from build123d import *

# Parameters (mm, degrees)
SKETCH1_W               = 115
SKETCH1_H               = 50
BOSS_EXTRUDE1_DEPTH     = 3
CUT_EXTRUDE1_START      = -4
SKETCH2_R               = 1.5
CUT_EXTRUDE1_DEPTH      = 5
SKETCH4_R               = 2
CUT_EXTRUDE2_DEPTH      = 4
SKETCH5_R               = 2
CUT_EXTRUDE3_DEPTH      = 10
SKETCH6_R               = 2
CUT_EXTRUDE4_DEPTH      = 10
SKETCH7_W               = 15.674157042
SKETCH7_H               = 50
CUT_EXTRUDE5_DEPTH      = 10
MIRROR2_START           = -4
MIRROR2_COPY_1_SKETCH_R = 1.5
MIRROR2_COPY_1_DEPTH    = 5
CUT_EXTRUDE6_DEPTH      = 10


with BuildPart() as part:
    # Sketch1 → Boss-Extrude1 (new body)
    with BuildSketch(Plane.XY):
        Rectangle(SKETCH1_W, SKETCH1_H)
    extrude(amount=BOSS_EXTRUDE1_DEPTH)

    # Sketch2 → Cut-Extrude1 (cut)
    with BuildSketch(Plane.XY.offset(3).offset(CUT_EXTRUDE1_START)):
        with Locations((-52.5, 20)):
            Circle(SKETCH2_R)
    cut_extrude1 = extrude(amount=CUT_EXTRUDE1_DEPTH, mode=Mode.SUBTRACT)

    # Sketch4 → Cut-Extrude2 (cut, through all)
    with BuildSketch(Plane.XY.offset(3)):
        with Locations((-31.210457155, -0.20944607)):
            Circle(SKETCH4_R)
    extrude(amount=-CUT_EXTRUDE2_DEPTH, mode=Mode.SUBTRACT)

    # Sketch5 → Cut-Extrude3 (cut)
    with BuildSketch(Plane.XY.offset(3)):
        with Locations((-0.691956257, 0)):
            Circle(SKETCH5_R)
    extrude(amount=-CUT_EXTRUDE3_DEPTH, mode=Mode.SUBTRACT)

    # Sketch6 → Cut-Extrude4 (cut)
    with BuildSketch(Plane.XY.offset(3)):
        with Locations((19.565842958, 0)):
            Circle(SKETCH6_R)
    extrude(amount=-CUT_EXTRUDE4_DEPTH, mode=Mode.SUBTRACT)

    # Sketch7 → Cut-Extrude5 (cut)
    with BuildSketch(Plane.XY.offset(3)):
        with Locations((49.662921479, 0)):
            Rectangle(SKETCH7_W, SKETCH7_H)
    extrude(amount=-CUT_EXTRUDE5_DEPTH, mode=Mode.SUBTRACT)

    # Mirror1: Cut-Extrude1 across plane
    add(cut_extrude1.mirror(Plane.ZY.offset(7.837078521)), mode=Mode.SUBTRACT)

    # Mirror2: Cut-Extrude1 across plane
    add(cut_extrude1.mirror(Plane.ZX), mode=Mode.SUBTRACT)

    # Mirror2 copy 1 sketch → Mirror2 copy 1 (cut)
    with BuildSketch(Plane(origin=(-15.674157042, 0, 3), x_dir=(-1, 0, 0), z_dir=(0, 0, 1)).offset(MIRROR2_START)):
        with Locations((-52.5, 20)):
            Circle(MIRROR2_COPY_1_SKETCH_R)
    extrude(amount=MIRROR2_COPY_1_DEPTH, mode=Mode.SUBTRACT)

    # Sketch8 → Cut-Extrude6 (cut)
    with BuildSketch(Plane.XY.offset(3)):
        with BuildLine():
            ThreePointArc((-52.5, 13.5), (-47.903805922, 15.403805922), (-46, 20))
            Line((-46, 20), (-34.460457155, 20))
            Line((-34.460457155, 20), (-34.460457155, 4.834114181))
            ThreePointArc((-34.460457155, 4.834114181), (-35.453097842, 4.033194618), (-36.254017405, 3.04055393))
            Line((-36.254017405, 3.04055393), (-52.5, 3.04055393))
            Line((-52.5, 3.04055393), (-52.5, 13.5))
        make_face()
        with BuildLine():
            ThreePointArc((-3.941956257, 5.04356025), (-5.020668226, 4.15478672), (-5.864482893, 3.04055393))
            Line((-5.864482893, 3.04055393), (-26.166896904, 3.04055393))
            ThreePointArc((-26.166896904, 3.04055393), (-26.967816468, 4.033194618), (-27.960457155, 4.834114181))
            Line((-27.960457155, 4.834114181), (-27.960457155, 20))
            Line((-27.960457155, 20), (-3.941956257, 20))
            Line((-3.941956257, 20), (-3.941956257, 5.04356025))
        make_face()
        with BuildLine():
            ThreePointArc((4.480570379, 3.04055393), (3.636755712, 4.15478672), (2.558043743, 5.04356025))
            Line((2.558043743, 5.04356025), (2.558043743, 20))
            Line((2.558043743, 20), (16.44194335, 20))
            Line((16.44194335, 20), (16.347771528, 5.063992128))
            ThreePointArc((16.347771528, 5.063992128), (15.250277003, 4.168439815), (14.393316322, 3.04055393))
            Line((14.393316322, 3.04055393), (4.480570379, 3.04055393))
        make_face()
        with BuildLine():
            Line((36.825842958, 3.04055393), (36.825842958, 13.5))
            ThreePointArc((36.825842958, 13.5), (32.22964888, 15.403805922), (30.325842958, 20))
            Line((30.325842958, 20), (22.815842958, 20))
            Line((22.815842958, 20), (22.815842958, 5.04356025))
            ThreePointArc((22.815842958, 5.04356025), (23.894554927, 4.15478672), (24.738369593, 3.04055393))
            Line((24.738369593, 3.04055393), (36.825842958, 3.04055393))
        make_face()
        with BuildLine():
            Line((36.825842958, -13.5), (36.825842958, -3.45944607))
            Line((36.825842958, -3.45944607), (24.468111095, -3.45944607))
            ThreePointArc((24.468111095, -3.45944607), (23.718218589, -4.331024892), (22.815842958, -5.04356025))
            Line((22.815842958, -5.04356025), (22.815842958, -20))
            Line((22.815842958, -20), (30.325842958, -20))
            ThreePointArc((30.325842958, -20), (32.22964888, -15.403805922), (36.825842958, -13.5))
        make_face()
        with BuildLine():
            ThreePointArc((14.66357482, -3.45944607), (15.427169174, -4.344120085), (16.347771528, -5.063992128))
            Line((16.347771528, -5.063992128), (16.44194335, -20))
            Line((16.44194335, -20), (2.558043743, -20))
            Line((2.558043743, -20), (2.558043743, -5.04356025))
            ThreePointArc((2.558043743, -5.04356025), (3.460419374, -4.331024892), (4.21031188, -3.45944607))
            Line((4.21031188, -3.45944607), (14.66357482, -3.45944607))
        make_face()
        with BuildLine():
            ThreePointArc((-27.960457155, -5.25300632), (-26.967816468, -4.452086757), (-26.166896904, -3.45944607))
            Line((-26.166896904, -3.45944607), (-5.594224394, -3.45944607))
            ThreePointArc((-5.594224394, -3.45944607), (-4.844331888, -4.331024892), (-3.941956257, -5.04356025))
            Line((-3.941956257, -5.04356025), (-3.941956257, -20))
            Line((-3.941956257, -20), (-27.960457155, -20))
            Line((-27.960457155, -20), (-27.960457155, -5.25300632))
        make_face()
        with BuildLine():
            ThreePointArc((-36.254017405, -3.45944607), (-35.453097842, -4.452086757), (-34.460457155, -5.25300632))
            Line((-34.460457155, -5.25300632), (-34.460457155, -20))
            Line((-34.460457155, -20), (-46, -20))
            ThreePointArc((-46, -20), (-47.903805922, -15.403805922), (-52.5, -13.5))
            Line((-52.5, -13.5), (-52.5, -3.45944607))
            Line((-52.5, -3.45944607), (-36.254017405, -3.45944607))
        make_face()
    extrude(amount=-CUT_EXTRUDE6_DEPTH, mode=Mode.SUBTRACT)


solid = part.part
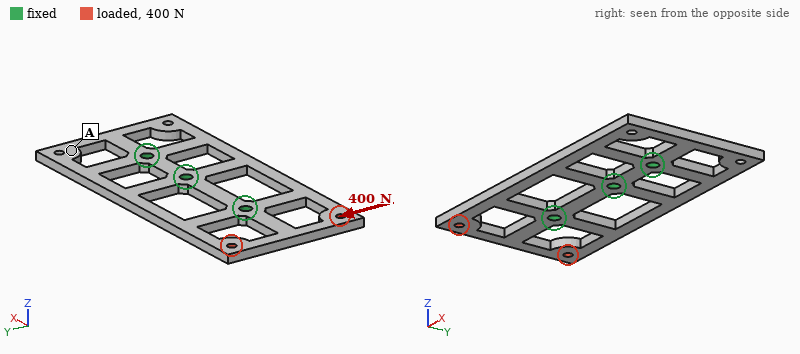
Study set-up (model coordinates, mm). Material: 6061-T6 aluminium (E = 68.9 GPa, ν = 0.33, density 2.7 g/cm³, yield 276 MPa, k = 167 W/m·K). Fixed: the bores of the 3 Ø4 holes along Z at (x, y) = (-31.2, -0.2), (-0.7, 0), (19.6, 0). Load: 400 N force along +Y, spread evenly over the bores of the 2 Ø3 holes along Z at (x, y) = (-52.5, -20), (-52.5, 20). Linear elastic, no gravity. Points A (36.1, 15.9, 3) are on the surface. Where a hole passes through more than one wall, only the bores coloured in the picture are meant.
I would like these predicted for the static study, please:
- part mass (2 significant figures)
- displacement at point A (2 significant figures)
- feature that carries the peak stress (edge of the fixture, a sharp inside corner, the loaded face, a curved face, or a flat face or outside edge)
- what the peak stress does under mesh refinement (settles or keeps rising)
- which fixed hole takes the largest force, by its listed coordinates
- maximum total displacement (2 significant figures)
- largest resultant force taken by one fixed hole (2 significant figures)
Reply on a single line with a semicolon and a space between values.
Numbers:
22 g; 12 µm; a sharp inside corner; keeps rising; (-31.2, -0.2); 61 µm; 480 N
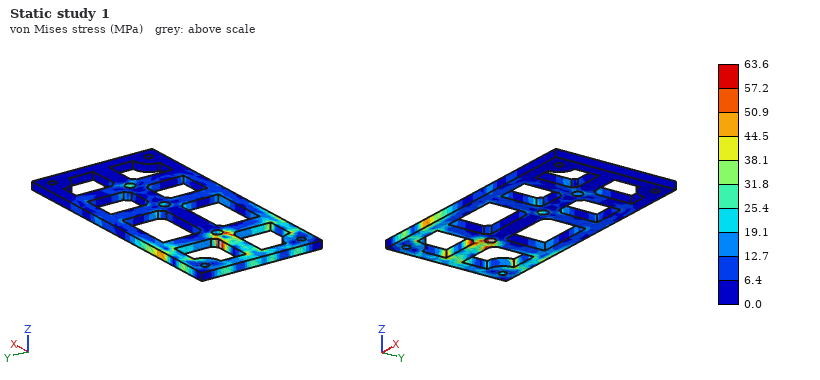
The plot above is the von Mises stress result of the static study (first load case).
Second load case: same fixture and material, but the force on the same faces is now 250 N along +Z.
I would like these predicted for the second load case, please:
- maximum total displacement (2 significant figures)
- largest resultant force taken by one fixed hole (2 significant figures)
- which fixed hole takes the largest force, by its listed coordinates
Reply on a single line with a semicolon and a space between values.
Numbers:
0.71 mm; 290 N; (-31.2, -0.2)
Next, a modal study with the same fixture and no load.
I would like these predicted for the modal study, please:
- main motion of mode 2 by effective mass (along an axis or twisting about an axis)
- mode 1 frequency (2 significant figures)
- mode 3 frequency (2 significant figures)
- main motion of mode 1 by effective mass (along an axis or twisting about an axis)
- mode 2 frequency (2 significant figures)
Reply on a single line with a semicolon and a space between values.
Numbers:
twisting about X; 2000 Hz; 2500 Hz; along Z; 2100 Hz
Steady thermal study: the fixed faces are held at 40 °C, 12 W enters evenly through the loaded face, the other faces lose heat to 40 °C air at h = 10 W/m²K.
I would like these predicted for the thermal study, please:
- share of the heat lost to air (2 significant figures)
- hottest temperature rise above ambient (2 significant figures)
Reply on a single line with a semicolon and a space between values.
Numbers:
6.3 %; 43 K
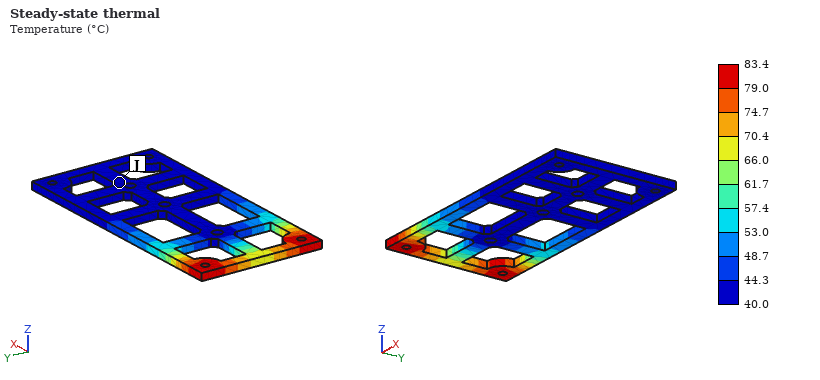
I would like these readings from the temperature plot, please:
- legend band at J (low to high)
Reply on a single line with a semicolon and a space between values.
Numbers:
40.0 to 44.3 °C
